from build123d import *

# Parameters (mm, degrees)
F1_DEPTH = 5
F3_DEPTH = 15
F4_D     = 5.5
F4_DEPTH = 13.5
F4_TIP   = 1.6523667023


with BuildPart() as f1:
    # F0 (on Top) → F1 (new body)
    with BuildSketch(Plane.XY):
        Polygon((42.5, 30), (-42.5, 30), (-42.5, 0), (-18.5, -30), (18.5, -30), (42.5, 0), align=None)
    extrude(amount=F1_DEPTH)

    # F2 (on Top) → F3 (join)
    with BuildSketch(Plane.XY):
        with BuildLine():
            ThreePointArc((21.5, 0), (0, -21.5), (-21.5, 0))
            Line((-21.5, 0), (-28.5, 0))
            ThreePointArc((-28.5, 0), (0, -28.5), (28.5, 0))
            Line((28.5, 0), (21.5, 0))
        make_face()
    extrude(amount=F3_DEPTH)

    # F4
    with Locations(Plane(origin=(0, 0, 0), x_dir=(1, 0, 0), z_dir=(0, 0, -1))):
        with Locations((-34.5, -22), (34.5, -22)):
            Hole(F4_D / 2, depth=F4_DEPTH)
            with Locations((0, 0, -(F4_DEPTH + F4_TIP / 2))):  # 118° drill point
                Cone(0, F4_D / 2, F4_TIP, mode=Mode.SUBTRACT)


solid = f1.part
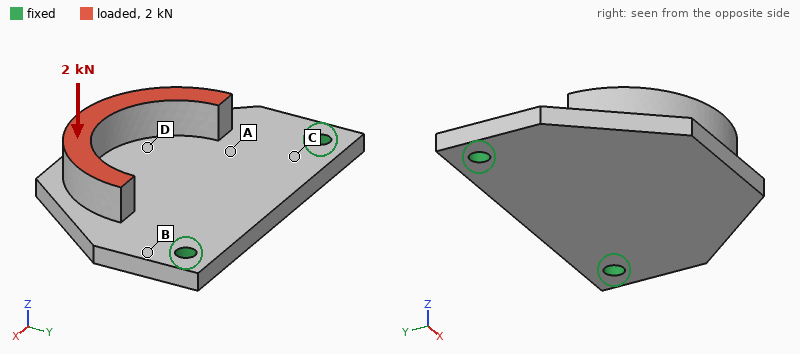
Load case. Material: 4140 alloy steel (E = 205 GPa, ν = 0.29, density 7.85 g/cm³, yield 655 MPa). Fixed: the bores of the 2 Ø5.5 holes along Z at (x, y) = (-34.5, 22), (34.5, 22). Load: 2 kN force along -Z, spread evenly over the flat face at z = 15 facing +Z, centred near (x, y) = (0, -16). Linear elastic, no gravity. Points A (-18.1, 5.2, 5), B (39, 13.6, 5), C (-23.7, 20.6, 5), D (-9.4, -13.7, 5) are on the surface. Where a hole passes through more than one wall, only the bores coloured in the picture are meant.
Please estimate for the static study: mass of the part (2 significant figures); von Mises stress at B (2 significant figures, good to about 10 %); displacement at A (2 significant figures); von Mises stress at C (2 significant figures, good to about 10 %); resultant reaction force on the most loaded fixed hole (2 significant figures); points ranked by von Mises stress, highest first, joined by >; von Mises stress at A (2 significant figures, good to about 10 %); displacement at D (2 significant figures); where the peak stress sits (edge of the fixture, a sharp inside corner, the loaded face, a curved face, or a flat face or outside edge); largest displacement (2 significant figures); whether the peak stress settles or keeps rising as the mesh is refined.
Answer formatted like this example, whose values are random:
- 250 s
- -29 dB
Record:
- 210 g
- 270 MPa
- 0.11 mm
- 180 MPa
- 1.0 kN
- B > C > A > D
- 110 MPa
- 0.29 mm
- edge of the fixture
- 0.47 mm
- keeps rising
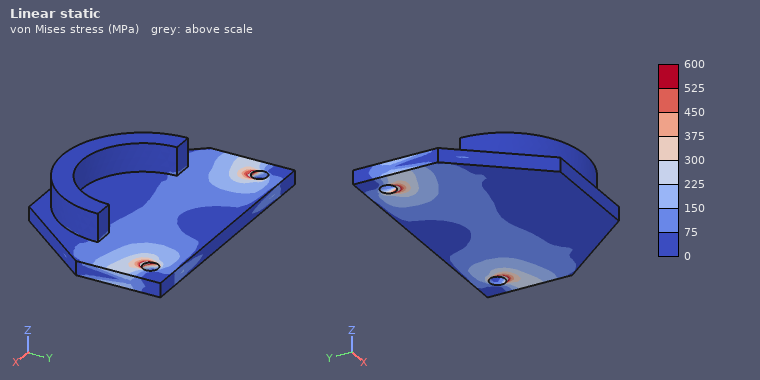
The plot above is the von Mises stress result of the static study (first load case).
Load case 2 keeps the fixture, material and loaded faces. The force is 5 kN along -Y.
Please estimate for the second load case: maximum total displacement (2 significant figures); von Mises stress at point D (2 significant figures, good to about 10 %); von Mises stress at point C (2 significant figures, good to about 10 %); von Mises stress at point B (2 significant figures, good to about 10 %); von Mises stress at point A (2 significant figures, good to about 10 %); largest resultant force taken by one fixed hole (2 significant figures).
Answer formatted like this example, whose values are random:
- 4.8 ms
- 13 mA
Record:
- 0.53 mm
- 67 MPa
- 180 MPa
- 270 MPa
- 180 MPa
- 2.7 kN
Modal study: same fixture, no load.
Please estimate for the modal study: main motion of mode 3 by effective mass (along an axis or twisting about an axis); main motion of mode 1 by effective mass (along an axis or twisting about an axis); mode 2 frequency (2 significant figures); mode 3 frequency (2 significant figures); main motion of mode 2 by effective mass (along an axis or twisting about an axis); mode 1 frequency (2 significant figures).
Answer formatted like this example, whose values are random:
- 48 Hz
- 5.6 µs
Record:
- along Z
- along Z
- 4500 Hz
- 5900 Hz
- twisting about Y
- 1200 Hz
